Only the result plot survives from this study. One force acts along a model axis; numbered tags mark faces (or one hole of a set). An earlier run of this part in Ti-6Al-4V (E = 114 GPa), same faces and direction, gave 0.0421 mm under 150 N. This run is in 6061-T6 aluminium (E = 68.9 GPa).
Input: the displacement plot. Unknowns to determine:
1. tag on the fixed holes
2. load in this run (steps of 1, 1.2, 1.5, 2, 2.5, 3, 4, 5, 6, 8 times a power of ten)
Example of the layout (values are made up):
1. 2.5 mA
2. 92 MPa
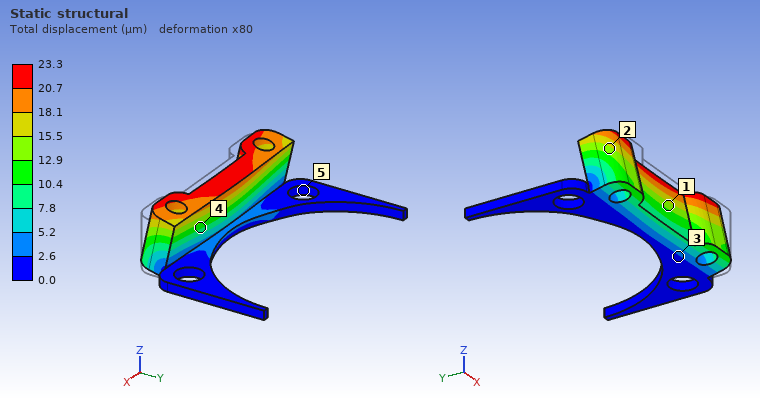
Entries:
1. 5
2. 50 N
